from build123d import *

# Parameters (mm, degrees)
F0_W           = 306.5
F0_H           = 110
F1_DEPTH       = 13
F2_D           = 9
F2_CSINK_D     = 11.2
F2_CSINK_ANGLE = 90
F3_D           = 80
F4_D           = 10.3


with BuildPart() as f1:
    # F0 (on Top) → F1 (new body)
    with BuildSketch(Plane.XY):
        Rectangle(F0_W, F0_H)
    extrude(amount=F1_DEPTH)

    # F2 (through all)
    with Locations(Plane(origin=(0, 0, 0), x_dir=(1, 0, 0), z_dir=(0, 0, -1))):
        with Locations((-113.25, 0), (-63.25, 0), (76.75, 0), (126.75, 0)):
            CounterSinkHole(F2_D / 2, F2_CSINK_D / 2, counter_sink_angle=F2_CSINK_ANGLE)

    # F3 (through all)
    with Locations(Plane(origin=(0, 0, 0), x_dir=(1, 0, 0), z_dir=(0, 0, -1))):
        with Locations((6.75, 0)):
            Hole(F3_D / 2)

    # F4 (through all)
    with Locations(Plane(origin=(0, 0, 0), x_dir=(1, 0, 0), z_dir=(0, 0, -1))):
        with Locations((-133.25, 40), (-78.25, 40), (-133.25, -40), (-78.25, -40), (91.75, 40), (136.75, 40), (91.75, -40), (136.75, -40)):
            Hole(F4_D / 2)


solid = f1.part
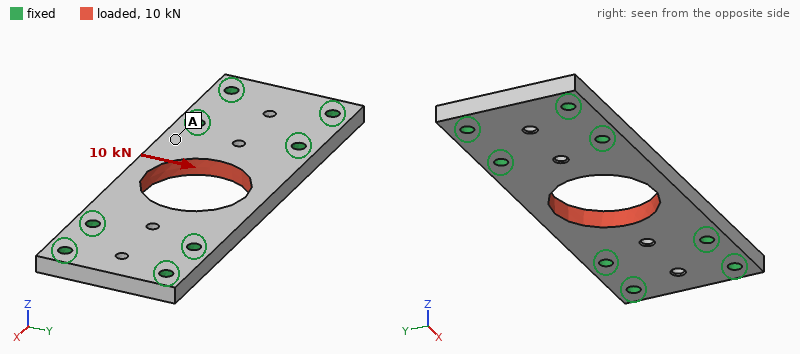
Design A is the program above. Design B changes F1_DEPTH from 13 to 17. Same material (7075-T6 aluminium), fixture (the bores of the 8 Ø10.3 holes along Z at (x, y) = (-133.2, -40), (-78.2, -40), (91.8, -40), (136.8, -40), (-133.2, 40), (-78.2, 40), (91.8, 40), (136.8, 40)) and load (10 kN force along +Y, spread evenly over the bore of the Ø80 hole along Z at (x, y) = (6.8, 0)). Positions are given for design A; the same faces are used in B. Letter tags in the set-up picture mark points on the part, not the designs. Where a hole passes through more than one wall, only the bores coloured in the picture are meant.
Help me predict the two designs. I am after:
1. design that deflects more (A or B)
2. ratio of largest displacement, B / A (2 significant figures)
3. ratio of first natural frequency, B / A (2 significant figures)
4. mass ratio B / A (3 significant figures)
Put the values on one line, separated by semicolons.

A; 0.76; 1.3; 1.31
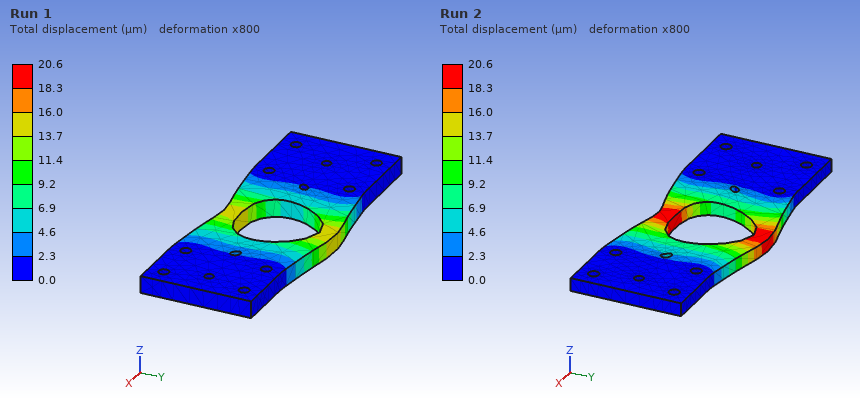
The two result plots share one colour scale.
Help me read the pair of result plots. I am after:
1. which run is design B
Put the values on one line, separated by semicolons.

Run 1
